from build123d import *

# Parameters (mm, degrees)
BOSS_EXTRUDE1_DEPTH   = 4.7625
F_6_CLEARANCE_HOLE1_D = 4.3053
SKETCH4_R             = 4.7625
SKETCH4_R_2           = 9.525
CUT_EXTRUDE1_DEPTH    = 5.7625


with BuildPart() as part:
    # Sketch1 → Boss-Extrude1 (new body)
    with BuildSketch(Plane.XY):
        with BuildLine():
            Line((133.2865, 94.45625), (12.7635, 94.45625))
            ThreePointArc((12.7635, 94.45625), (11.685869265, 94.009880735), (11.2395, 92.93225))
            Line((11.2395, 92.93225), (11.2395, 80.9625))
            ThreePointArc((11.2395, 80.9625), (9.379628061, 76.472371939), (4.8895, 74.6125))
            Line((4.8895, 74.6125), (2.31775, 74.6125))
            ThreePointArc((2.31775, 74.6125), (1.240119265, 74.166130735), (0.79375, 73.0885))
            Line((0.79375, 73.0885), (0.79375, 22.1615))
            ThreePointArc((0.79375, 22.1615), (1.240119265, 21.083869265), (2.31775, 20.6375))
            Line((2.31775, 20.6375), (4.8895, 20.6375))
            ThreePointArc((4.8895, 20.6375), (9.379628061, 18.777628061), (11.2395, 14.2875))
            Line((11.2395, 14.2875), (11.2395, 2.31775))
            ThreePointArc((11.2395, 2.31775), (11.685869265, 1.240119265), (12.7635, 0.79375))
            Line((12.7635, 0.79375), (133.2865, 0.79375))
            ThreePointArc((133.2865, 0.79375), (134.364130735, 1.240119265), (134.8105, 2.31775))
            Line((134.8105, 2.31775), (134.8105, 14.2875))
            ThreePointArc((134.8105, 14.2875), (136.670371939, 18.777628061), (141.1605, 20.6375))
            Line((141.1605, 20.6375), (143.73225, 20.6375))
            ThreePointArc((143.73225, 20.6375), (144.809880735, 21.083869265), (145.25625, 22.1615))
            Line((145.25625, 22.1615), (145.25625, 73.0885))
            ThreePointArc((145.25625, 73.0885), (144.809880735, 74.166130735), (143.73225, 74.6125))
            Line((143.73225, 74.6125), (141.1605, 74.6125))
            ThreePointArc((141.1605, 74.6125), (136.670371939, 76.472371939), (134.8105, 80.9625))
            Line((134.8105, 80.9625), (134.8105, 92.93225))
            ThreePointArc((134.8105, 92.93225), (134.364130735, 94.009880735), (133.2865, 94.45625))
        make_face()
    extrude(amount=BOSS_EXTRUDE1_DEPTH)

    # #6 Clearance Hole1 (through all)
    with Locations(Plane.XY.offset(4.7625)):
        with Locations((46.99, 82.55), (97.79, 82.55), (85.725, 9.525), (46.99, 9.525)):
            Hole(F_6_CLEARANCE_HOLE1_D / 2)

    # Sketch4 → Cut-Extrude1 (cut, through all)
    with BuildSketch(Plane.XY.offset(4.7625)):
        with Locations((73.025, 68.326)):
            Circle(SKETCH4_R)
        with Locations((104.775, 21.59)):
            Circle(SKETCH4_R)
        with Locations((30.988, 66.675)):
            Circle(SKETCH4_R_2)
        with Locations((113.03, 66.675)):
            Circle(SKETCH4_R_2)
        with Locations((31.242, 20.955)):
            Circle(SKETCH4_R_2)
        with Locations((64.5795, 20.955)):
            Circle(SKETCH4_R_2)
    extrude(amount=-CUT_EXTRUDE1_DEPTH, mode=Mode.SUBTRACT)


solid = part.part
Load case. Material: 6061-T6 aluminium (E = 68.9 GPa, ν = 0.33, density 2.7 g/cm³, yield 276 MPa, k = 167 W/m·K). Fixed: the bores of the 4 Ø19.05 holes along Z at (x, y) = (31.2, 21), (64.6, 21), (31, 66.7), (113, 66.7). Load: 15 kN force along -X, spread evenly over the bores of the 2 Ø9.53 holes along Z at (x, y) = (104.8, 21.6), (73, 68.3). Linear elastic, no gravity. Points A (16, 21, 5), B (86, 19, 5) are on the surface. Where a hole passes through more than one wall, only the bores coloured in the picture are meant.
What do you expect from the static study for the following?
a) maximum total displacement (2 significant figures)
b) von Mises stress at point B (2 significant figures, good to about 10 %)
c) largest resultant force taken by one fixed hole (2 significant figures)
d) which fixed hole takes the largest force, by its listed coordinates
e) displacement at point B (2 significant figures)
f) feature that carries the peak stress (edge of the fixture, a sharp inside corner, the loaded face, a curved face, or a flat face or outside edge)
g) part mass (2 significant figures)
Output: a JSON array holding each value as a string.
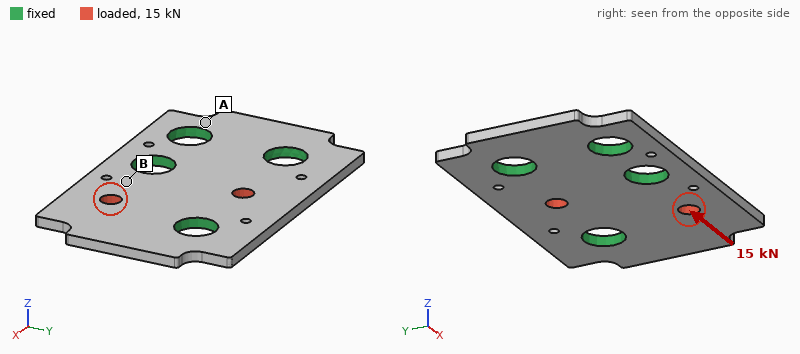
["27 µm", "49 MPa", "5.7 kN", "(64.6, 21)", "8.4 µm", "a curved face", "150 g"]
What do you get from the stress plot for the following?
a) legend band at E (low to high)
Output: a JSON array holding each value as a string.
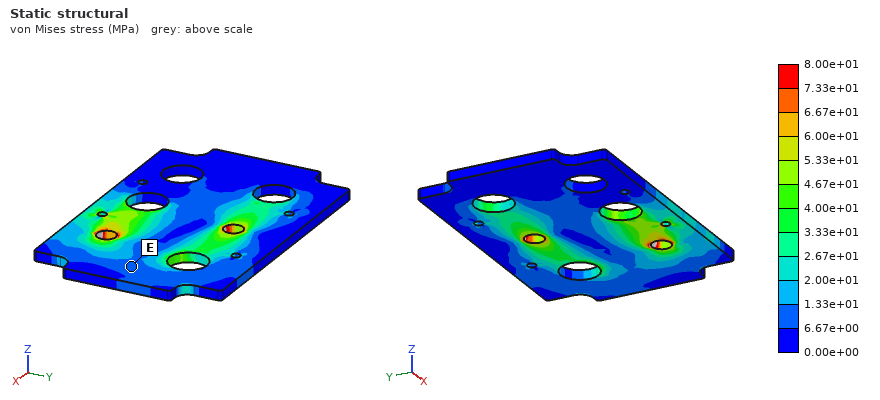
["6.67e+00 to 1.33e+01 MPa"]
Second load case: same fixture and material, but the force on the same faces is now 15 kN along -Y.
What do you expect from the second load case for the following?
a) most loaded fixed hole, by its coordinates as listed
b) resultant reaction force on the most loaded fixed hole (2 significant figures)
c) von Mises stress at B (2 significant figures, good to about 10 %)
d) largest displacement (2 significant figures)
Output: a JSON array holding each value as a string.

["(113, 66.7)", "7.6 kN", "23 MPa", "30 µm"]
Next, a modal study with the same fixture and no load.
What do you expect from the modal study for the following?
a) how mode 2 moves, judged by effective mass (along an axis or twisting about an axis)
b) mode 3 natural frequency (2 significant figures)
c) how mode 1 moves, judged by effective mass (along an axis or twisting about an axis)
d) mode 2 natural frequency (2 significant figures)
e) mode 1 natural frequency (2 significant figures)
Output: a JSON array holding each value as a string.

["along Z", "4800 Hz", "along Z", "4500 Hz", "1900 Hz"]
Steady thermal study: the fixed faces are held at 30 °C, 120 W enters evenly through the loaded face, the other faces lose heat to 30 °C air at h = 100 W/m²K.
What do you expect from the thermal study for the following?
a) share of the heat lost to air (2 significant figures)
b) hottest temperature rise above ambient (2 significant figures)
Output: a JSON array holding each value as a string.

["18 %", "39 K"]
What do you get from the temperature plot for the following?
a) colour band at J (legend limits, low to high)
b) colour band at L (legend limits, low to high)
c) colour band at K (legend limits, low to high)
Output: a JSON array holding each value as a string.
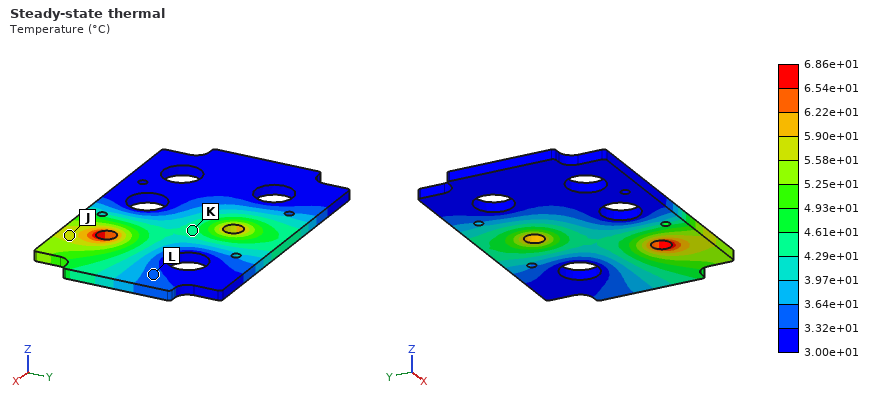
["5.58e+01 to 5.90e+01 °C", "3.32e+01 to 3.64e+01 °C", "4.29e+01 to 4.61e+01 °C"]
